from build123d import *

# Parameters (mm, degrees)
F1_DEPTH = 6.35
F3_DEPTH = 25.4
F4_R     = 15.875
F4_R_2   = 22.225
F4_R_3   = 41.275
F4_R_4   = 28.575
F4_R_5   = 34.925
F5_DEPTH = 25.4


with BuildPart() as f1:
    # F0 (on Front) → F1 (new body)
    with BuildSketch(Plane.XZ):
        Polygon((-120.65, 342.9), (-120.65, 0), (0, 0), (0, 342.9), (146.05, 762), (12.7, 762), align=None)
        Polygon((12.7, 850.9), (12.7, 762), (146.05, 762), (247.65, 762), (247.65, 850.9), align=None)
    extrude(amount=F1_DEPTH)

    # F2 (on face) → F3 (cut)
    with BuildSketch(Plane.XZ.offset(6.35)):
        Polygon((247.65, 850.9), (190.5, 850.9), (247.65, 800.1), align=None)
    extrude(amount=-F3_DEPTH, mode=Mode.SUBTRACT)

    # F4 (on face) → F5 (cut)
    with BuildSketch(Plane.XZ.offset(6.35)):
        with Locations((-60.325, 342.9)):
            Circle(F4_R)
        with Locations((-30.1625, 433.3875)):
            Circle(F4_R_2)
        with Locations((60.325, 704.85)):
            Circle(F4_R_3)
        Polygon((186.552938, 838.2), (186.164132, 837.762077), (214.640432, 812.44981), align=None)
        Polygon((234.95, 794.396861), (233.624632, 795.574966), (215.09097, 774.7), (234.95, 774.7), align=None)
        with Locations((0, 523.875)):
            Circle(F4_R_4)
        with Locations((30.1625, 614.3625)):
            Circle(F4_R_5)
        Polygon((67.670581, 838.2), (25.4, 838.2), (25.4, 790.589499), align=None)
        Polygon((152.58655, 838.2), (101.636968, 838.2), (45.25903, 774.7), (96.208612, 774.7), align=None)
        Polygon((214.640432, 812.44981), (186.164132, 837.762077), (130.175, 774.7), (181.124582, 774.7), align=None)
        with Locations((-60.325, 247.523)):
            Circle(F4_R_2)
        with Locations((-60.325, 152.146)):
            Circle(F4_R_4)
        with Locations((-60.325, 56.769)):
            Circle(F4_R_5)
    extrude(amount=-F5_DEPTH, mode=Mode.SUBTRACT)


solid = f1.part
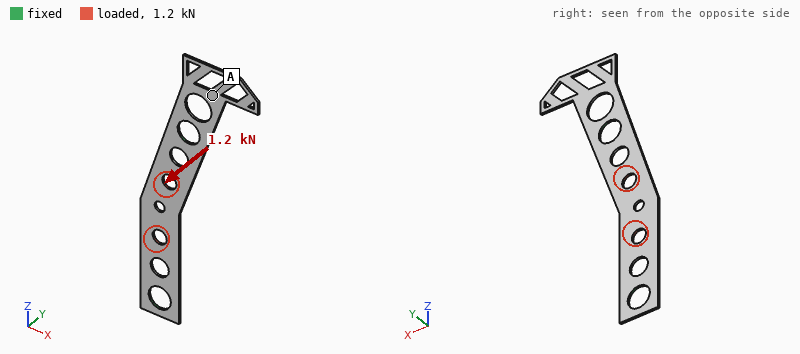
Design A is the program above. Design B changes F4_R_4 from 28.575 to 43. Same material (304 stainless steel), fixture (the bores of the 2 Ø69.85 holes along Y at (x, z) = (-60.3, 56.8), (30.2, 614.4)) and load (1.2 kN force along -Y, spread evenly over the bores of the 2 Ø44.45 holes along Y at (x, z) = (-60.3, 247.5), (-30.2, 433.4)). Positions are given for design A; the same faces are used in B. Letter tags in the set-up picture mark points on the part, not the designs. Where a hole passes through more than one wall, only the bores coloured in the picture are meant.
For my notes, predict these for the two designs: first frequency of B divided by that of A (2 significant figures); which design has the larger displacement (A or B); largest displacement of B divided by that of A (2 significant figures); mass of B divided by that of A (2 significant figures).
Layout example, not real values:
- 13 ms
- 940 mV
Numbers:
- 1.00
- B
- 1.3
- 0.92
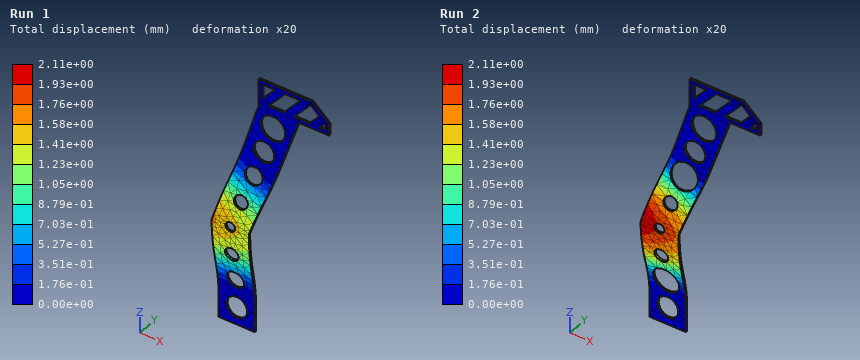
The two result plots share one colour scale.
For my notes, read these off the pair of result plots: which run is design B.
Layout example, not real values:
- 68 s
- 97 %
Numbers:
- Run 2
